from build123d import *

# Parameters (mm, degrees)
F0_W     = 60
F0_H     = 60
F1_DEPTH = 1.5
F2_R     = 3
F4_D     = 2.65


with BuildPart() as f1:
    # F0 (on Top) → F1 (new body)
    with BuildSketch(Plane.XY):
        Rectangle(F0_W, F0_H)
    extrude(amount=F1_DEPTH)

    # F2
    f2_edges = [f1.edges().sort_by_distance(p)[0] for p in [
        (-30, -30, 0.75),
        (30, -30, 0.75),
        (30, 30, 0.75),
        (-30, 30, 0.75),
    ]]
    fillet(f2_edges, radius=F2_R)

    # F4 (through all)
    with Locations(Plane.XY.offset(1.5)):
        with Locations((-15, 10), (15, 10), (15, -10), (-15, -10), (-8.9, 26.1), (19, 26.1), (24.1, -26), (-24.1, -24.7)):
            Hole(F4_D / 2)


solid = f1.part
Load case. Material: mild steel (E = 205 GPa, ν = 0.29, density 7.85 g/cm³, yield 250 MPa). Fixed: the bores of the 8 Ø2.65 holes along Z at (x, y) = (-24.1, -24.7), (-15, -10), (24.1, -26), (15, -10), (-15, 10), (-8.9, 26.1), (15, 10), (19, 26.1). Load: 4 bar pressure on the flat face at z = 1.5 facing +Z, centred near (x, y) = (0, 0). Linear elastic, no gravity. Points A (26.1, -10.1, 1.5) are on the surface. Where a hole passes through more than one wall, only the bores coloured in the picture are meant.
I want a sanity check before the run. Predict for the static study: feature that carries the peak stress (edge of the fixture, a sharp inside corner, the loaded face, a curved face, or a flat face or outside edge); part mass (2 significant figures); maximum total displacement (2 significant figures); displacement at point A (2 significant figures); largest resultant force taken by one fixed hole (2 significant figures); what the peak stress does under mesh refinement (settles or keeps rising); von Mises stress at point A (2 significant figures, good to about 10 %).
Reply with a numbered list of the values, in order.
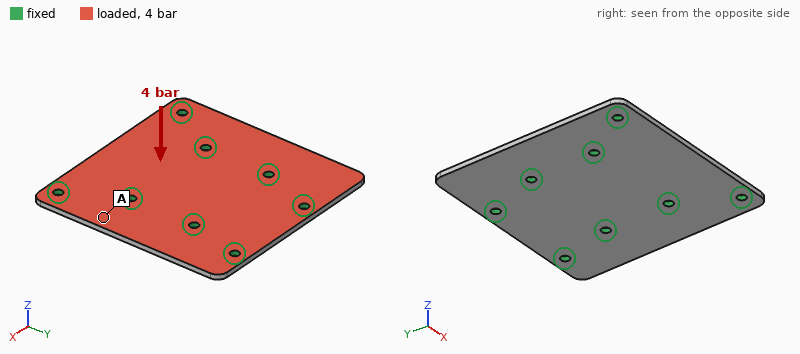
1. edge of the fixture
2. 42 g
3. 81 µm
4. 14 µm
5. 240 N
6. keeps rising
7. 21 MPa
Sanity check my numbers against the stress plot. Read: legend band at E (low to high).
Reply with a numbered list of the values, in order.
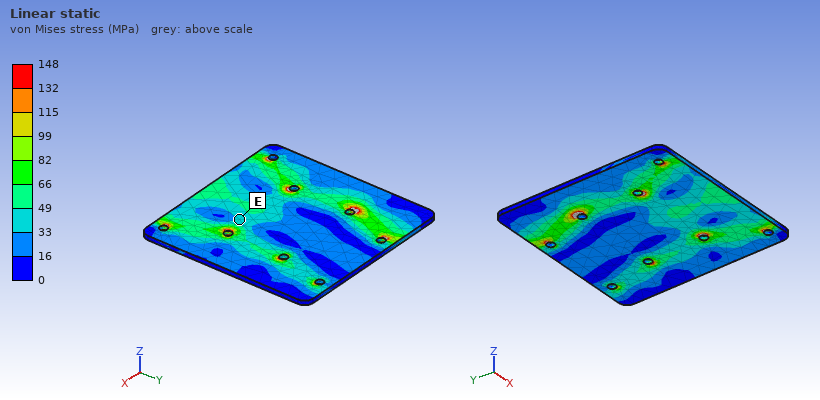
1. 33 to 49 MPa
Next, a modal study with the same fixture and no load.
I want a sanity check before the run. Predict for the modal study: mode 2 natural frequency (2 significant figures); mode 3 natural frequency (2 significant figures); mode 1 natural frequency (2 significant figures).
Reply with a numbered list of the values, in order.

1. 4900 Hz
2. 6500 Hz
3. 4400 Hz
